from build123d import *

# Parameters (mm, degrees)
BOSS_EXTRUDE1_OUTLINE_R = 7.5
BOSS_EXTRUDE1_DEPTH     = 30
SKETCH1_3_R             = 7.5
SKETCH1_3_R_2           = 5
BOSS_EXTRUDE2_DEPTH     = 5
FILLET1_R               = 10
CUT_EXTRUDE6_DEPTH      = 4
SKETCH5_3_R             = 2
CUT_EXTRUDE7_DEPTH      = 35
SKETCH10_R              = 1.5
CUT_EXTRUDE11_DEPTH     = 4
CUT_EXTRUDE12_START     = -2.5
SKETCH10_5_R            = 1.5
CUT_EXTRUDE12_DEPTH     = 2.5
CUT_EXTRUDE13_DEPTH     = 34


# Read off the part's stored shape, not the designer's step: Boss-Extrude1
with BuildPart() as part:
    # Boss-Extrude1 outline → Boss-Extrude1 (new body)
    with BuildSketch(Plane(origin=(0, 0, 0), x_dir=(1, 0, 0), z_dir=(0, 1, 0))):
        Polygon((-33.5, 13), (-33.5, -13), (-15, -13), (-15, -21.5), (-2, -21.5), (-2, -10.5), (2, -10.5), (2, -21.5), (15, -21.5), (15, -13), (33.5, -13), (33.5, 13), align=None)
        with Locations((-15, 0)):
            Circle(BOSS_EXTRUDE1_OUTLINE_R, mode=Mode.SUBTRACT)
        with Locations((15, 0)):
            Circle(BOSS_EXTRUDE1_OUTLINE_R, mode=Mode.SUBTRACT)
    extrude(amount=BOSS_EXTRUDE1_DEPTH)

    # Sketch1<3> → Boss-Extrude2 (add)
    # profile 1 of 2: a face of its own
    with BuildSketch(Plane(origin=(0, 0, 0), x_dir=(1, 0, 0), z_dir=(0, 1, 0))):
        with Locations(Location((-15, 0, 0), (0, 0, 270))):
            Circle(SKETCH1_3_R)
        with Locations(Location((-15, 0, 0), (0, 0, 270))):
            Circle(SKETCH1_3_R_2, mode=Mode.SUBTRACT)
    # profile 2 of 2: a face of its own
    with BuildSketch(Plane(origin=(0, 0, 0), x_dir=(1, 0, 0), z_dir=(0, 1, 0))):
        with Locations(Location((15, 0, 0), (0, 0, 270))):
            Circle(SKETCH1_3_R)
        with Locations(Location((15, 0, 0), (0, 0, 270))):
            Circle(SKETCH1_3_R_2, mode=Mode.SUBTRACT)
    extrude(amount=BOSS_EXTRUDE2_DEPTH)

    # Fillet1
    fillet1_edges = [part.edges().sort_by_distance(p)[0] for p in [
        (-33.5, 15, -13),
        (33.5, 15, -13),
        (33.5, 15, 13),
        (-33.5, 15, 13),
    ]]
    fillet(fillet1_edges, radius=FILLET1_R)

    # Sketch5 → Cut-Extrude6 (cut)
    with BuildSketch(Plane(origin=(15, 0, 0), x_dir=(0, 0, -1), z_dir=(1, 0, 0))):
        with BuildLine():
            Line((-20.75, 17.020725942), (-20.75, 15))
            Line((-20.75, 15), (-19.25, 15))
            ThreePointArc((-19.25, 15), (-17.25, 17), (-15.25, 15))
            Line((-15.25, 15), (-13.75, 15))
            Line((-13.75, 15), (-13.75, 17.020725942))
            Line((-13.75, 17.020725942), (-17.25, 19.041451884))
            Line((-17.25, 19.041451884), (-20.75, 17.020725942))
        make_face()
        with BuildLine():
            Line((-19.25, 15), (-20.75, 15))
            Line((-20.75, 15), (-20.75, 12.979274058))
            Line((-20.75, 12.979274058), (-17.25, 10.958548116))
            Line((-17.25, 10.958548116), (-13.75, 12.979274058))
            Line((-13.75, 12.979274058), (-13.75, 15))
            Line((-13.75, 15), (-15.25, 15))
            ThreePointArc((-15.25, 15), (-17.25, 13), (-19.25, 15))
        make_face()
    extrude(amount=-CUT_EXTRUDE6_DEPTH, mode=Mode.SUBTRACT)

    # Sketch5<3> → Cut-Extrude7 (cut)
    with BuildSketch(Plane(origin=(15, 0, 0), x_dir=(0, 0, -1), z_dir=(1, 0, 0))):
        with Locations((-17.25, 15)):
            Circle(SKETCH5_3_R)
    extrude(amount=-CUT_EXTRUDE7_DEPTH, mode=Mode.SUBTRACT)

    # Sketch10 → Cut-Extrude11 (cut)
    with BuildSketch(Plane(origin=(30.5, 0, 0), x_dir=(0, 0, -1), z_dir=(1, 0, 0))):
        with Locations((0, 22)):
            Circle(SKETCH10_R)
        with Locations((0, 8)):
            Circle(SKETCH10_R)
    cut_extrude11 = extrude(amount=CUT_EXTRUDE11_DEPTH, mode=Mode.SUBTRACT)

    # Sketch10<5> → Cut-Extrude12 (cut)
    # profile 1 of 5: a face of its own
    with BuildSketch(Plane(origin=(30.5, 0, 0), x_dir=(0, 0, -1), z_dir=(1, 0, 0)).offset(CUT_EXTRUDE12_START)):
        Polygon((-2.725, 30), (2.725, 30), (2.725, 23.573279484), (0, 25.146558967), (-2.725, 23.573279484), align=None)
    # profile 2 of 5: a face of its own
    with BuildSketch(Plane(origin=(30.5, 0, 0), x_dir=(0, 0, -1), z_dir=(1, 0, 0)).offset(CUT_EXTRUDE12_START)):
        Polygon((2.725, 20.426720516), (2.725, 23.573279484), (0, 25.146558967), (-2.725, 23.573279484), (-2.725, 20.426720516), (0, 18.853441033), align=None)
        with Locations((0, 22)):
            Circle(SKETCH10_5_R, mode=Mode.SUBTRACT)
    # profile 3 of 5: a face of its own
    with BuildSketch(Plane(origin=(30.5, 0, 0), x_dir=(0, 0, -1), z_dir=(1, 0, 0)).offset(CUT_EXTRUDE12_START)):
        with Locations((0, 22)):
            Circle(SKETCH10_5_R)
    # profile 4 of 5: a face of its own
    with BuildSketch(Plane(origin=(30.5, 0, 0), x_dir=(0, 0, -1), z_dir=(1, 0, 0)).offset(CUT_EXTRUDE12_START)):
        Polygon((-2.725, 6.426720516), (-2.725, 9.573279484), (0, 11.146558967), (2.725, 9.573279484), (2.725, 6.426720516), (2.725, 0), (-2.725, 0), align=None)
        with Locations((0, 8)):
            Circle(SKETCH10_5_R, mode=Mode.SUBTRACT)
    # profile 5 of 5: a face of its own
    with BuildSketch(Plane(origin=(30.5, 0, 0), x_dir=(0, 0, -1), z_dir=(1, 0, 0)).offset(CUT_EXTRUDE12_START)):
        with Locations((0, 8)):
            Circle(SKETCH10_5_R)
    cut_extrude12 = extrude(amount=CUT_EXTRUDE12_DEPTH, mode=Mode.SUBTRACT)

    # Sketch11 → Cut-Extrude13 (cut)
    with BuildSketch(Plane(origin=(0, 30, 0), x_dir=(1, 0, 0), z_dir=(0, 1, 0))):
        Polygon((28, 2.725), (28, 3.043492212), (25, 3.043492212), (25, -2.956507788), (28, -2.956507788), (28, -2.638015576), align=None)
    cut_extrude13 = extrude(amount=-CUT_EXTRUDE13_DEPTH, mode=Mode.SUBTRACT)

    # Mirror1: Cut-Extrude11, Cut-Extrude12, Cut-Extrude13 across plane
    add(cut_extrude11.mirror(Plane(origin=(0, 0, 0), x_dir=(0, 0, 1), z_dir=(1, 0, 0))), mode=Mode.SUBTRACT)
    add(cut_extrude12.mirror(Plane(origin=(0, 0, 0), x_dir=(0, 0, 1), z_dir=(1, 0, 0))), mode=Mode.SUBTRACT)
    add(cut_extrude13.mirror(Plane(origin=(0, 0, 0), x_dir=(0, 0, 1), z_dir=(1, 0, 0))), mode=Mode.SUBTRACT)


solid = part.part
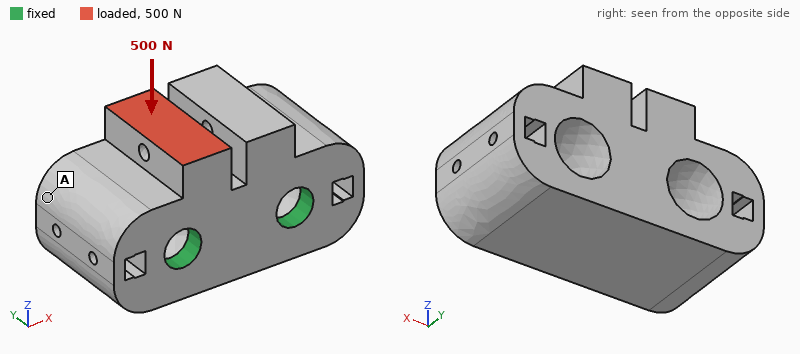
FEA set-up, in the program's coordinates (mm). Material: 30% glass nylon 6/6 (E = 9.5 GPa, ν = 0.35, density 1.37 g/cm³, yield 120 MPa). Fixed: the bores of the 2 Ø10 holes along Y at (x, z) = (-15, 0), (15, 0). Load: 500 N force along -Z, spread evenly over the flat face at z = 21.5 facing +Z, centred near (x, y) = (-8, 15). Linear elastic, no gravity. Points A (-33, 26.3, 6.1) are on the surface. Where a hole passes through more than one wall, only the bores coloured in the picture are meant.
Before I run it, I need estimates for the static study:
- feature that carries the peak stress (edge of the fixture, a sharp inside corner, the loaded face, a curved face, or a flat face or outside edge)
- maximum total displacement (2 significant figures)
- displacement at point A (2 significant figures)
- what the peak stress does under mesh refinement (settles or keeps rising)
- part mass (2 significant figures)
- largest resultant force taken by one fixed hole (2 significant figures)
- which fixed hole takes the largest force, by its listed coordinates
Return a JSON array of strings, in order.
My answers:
["edge of the fixture", "46 µm", "29 µm", "keeps rising", "61 g", "370 N", "(-15, 0)"]
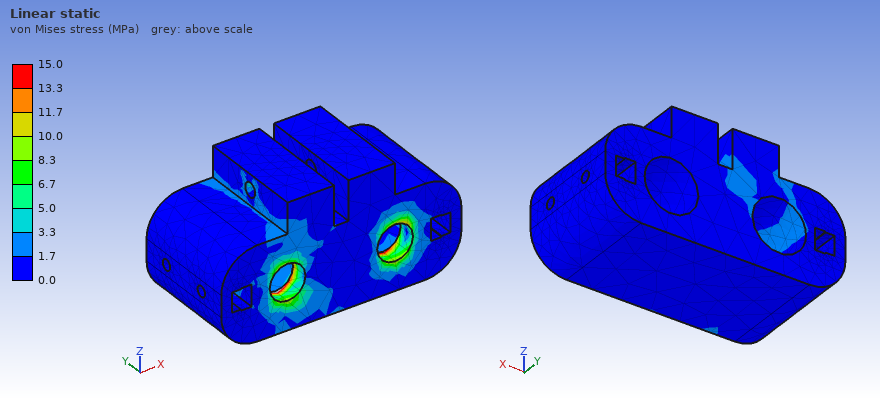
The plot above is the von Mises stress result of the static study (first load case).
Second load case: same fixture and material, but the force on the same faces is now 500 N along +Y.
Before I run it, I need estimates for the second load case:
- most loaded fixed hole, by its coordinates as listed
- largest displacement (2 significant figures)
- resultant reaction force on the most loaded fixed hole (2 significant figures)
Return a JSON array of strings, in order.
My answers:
["(-15, 0)", "80 µm", "400 N"]
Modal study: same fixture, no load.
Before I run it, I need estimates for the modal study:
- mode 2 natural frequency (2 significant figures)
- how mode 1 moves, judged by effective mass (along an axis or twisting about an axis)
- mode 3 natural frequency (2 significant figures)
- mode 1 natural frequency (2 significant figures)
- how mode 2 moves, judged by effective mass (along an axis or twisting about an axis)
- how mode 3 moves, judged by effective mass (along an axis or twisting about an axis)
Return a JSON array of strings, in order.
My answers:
["5400 Hz", "along Z", "6100 Hz", "2800 Hz", "along X", "twisting about Y"]
